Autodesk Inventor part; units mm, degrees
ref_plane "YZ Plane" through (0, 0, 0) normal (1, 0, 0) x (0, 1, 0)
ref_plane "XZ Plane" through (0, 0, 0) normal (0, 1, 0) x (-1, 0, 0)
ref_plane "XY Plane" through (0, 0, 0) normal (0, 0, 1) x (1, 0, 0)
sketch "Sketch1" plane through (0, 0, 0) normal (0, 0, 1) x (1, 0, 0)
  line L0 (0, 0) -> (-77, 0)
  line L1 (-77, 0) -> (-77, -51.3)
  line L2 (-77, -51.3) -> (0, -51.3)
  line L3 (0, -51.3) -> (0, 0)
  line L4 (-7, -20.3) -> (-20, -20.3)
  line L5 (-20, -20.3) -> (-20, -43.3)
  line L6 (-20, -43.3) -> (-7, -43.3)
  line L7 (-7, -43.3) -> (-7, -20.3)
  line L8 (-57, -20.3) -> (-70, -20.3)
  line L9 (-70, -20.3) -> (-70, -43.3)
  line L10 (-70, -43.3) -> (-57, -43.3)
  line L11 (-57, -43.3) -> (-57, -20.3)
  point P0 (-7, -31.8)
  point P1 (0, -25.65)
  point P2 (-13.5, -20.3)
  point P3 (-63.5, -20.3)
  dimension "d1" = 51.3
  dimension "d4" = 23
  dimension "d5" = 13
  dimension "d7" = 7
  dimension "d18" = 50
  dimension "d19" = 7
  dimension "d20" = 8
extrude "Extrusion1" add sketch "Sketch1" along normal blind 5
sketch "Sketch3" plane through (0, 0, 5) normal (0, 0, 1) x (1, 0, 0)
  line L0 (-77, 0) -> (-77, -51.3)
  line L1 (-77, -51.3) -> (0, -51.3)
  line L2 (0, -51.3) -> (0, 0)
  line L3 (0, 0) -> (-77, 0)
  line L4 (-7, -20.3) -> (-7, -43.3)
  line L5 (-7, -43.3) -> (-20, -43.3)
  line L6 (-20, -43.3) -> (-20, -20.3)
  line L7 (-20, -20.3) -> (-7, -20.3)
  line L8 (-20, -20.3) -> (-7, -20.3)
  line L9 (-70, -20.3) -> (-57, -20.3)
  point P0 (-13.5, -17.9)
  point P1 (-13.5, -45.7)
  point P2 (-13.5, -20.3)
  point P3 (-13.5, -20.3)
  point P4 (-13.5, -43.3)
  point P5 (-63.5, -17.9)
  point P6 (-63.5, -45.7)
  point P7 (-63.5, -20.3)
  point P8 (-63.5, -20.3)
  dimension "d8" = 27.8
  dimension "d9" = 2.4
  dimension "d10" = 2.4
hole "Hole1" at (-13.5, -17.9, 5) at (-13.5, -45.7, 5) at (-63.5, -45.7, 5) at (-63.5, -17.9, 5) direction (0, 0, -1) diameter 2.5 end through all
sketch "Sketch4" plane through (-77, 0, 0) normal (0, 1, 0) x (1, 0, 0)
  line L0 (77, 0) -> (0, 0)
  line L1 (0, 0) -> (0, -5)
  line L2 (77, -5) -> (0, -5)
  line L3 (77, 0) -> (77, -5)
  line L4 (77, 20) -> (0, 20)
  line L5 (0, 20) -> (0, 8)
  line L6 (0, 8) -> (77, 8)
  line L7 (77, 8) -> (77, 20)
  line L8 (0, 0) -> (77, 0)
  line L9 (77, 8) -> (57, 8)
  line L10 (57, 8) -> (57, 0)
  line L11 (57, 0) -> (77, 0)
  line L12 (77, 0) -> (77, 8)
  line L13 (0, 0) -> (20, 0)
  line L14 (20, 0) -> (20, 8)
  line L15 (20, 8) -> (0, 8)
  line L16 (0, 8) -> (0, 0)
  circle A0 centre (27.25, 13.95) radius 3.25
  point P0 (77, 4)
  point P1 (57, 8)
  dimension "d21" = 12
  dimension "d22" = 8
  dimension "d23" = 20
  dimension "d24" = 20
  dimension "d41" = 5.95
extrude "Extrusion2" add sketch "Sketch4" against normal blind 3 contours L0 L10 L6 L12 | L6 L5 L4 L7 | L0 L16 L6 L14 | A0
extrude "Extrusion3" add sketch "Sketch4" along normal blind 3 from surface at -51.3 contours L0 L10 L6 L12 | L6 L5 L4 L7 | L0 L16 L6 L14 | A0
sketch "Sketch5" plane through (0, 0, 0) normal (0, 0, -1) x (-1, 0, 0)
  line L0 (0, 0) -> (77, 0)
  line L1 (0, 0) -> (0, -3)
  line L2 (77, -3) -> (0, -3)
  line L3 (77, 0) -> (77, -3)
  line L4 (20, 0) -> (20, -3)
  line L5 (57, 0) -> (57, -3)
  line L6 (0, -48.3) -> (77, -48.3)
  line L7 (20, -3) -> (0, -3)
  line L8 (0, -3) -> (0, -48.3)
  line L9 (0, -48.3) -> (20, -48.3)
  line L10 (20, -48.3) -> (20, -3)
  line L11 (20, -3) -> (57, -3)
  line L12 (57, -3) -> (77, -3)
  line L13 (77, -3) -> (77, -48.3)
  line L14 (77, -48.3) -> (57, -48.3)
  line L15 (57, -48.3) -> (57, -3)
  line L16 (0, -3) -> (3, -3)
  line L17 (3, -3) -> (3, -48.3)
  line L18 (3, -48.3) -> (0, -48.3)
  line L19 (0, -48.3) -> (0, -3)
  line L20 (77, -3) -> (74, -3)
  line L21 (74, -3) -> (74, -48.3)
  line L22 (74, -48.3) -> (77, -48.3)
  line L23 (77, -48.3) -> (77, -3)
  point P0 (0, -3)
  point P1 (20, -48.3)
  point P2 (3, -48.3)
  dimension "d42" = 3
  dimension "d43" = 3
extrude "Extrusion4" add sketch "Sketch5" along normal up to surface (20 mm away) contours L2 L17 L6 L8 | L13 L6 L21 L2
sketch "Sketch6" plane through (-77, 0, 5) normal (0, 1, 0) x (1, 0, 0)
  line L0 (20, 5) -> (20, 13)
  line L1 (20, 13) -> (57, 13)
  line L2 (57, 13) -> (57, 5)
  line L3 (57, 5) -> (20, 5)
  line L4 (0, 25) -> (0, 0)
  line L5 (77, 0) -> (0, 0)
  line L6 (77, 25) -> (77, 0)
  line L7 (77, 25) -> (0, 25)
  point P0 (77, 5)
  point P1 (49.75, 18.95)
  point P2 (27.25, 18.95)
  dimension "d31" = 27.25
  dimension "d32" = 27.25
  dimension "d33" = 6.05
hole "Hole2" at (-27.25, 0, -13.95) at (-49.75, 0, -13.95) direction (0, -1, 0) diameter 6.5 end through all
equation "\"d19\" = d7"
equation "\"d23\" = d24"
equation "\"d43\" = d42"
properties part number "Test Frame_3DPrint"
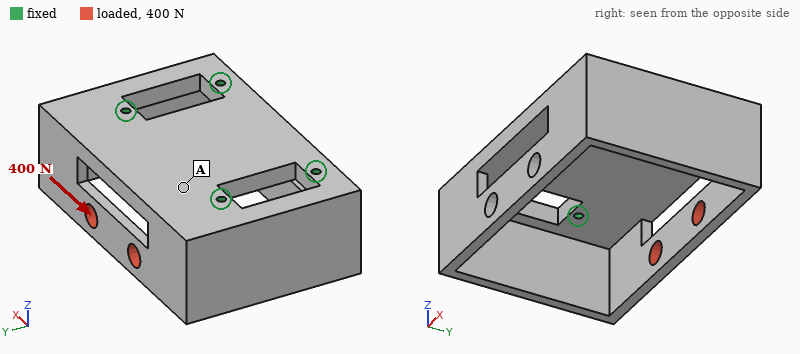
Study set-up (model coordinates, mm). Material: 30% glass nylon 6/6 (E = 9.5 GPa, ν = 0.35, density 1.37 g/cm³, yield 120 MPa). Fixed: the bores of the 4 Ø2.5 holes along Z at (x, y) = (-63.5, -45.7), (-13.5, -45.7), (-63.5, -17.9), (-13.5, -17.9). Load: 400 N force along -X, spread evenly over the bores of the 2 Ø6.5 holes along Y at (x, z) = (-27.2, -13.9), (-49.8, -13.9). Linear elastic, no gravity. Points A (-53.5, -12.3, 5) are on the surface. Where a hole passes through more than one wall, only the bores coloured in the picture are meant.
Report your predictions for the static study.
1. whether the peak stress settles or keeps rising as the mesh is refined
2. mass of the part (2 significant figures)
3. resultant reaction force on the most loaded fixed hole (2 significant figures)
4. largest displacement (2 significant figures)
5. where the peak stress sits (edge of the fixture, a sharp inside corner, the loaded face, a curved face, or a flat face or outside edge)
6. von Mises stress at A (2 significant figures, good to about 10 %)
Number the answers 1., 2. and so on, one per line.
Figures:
1. keeps rising
2. 40 g
3. 240 N
4. 0.16 mm
5. edge of the fixture
6. 4.7 MPa
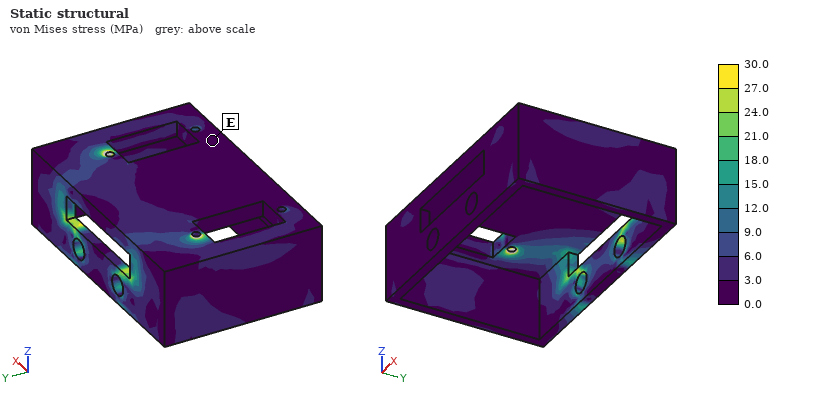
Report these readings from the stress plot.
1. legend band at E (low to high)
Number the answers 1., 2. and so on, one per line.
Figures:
1. 0.0 to 3.0 MPa
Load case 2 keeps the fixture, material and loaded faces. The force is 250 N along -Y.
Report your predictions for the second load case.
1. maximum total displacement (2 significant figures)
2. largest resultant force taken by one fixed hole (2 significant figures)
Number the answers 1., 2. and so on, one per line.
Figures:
1. 1.1 mm
2. 130 N
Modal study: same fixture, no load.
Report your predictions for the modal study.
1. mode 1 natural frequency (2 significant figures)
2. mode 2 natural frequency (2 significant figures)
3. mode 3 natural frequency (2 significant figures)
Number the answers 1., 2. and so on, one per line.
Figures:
1. 2100 Hz
2. 2100 Hz
3. 2700 Hz
